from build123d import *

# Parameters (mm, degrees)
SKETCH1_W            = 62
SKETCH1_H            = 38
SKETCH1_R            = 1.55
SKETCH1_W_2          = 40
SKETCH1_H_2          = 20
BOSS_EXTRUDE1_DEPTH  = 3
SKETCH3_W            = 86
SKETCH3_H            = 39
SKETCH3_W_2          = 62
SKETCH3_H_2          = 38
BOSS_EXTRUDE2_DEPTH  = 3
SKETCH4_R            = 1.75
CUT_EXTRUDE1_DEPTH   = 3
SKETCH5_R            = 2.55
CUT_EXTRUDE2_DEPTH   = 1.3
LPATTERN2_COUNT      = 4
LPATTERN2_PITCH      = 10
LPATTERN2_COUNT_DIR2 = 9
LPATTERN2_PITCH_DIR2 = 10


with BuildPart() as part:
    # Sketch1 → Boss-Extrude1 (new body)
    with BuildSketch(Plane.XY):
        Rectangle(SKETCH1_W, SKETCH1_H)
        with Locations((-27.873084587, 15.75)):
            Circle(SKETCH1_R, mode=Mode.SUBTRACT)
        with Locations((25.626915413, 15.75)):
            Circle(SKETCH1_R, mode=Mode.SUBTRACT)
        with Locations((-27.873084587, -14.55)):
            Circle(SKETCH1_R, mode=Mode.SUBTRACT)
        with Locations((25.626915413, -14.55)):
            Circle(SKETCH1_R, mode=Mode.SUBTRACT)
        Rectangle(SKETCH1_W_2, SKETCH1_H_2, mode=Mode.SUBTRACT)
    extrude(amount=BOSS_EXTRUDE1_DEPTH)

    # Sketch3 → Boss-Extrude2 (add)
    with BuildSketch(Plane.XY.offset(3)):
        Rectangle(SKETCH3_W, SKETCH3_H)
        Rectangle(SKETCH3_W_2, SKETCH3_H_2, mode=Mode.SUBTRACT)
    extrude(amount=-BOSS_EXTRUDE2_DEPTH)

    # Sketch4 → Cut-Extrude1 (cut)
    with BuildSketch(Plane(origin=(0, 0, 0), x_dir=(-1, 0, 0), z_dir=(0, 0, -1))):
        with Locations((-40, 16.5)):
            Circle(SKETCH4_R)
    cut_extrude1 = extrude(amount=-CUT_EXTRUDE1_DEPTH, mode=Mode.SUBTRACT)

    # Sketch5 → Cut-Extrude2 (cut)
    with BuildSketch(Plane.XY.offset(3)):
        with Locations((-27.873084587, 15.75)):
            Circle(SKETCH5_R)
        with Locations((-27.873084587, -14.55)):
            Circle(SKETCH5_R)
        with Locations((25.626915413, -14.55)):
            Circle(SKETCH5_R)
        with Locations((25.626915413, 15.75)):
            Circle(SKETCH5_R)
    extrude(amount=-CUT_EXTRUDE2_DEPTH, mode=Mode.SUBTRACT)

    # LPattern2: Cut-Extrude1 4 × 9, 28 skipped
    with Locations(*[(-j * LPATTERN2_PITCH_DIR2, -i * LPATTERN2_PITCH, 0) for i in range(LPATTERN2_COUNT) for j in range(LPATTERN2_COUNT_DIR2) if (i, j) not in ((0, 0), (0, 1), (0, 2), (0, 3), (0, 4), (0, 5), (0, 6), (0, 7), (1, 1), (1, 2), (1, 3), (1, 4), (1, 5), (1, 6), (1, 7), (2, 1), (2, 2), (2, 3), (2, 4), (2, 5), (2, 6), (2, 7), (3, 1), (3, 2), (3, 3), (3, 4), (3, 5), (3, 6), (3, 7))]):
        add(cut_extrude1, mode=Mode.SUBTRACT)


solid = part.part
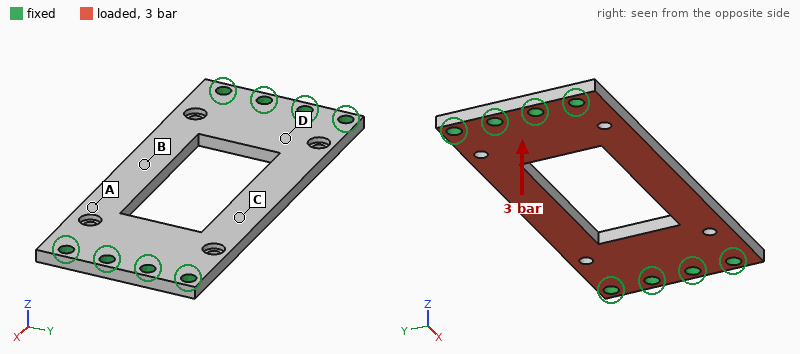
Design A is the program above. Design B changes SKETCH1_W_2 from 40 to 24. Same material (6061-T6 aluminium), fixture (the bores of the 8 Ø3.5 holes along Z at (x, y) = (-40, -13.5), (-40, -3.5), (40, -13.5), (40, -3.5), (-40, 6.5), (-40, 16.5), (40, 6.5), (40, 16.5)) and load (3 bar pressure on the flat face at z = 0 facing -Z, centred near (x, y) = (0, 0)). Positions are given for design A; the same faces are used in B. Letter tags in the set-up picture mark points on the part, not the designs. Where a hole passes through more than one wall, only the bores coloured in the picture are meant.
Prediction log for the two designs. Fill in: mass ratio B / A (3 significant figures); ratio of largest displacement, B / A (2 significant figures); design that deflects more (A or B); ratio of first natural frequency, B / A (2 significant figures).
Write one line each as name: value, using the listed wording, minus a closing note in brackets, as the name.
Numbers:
mass ratio B / A: 1.13
ratio of largest displacement, B / A: 1.2
design that deflects more: B
ratio of first natural frequency, B / A: 0.92
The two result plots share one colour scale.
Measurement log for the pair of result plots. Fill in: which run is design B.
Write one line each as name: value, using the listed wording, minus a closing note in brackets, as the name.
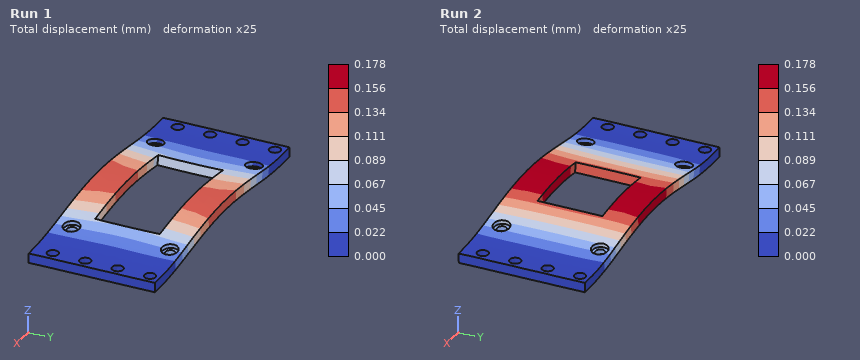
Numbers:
which run is design B: Run 2
